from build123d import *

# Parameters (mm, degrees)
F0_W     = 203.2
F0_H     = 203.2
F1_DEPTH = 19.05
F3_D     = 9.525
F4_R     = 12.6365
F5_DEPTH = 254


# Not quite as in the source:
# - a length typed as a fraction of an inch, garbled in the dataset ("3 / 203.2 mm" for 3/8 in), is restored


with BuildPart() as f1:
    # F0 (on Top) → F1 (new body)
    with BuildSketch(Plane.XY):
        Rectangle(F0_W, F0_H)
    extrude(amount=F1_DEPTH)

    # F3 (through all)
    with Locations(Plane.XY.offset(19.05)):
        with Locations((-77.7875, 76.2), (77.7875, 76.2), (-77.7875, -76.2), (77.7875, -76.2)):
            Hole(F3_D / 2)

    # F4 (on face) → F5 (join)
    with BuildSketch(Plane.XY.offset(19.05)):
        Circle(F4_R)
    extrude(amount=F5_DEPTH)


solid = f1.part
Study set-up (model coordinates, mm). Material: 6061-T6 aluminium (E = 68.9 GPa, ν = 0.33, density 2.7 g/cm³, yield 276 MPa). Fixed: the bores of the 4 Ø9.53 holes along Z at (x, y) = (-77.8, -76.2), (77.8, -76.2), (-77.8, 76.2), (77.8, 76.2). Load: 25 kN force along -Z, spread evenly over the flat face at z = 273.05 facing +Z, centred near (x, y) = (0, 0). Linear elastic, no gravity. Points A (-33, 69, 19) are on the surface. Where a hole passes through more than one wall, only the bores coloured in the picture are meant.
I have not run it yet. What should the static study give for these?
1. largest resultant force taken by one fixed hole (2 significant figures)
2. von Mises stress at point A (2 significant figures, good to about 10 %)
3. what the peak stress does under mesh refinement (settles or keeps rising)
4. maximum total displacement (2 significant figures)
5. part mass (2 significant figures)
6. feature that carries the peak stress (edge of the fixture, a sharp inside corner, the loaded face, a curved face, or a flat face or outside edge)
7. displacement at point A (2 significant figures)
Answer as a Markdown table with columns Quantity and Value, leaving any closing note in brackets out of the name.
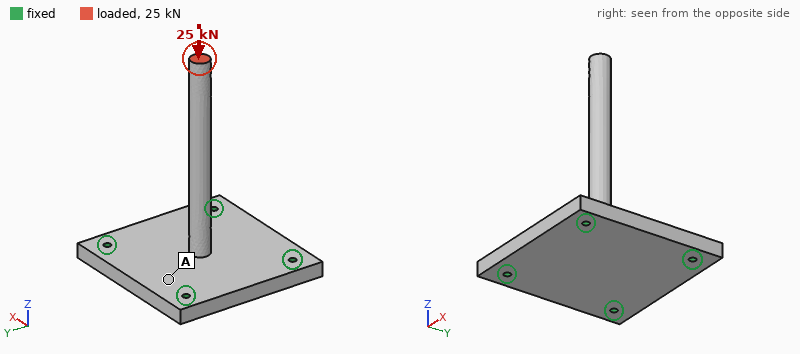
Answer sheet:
| Quantity | Value |
|---|---|
| largest resultant force taken by one fixed hole | 6.3 kN |
| von Mises stress at point A | 19 MPa |
| what the peak stress does under mesh refinement | keeps rising |
| maximum total displacement | 0.39 mm |
| part mass | 2.5 kg |
| feature that carries the peak stress | edge of the fixture |
| displacement at point A | 0.068 mm |
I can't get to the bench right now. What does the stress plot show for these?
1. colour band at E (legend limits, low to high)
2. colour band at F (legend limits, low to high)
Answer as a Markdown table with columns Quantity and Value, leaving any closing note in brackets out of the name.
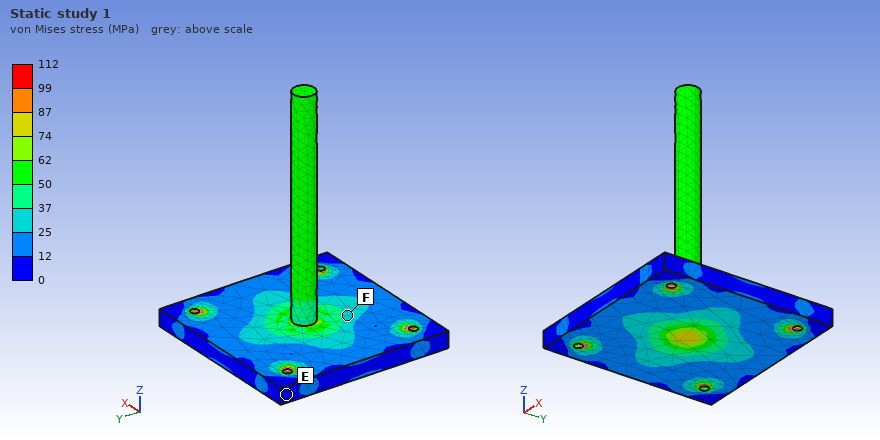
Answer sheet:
| Quantity | Value |
|---|---|
| colour band at E | 0 to 12 MPa |
| colour band at F | 25 to 37 MPa |
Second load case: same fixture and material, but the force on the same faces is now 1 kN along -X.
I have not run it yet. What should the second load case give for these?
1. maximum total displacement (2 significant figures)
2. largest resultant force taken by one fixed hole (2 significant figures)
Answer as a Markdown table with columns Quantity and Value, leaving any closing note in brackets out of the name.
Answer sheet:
| Quantity | Value |
|---|---|
| maximum total displacement | 4.4 mm |
| largest resultant force taken by one fixed hole | 1.0 kN |
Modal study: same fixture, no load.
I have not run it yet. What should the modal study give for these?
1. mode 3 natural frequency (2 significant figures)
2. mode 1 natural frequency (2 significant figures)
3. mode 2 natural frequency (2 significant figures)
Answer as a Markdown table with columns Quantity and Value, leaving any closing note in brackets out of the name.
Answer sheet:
| Quantity | Value |
|---|---|
| mode 3 natural frequency | 1600 Hz |
| mode 1 natural frequency | 260 Hz |
| mode 2 natural frequency | 260 Hz |
